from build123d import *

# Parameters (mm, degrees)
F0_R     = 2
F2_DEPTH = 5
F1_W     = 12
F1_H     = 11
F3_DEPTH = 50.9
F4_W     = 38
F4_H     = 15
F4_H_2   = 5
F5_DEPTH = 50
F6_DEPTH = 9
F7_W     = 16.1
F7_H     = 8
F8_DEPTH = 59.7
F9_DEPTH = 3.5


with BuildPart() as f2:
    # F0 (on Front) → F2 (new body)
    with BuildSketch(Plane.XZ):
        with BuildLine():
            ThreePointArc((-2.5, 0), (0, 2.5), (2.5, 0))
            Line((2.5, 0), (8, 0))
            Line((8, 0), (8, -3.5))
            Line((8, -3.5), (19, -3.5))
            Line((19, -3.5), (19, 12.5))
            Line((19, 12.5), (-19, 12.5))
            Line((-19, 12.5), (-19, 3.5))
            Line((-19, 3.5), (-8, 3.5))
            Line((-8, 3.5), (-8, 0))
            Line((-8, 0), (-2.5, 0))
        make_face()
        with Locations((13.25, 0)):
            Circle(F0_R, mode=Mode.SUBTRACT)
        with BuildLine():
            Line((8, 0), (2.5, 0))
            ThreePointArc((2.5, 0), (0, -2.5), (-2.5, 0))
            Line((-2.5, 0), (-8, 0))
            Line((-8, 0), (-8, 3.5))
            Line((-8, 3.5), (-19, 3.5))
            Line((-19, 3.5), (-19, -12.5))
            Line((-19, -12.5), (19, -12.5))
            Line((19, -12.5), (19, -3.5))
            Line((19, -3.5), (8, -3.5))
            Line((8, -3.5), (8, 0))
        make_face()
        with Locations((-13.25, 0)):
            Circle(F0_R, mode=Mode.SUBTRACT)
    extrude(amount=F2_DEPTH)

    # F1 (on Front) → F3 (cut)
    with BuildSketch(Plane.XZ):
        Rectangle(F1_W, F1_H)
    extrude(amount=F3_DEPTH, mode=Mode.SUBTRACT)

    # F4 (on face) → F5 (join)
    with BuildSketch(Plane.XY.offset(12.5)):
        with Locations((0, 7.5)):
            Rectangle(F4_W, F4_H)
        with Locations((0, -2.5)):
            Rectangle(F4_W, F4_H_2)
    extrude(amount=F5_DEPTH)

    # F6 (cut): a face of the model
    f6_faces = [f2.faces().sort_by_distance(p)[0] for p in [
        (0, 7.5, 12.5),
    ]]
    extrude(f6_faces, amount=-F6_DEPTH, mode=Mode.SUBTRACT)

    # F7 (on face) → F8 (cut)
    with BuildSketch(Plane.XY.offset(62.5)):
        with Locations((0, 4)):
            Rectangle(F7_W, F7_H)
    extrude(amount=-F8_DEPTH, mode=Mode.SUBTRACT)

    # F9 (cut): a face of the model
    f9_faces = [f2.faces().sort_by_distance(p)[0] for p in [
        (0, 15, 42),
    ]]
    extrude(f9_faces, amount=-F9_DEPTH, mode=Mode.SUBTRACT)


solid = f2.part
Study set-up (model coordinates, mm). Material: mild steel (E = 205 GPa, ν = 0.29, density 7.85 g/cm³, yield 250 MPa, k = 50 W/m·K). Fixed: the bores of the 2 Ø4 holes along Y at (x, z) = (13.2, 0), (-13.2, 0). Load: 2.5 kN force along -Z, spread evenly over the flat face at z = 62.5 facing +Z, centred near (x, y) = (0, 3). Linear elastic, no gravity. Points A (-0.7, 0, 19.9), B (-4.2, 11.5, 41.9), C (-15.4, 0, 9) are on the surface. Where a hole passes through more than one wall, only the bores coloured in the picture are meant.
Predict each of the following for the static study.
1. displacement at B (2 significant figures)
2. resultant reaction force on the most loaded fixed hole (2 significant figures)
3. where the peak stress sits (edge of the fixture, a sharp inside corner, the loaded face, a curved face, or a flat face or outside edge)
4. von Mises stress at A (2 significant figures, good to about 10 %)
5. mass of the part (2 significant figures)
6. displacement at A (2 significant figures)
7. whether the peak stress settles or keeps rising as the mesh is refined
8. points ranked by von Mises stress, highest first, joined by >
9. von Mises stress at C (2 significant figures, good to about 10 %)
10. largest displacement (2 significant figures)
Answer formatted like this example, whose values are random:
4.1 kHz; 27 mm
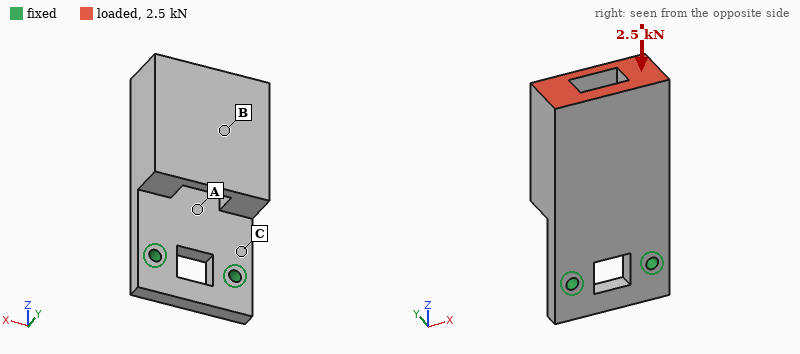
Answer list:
0.16 mm; 1.3 kN; edge of the fixture; 70 MPa; 200 g; 0.045 mm; keeps rising; C > A > B; 130 MPa; 0.25 mm
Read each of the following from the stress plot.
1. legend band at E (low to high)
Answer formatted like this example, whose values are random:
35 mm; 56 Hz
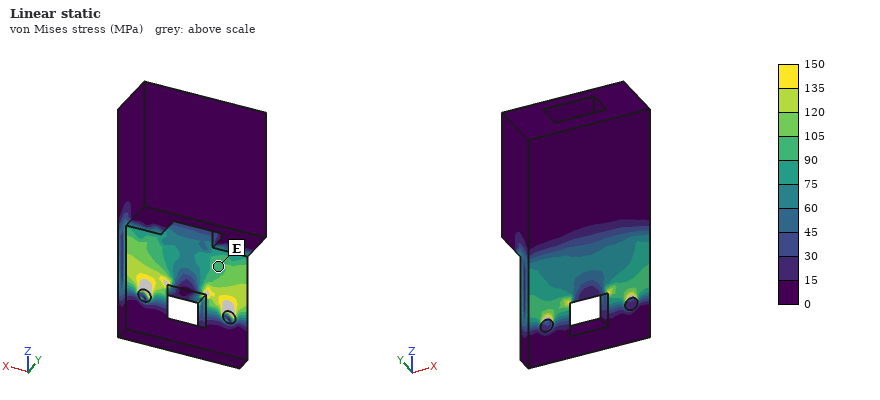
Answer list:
90 to 105 MPa
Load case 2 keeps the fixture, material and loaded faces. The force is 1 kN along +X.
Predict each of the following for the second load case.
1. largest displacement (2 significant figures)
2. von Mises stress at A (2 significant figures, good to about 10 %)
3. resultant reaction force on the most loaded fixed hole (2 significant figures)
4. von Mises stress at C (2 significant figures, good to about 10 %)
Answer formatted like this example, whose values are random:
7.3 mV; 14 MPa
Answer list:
27 µm; 21 MPa; 2.3 kN; 35 MPa
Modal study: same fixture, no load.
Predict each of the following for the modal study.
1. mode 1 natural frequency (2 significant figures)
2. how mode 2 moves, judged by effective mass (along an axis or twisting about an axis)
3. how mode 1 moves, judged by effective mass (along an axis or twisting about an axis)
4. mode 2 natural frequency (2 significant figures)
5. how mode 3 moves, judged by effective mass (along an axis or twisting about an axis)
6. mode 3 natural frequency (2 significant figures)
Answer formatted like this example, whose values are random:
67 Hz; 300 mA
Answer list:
620 Hz; along X; along Y; 2800 Hz; along X; 4200 Hz
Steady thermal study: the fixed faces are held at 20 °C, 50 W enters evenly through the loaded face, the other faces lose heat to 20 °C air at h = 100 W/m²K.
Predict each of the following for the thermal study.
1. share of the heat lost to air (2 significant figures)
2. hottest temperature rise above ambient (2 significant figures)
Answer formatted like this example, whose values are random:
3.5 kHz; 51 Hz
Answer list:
79 %; 85 K
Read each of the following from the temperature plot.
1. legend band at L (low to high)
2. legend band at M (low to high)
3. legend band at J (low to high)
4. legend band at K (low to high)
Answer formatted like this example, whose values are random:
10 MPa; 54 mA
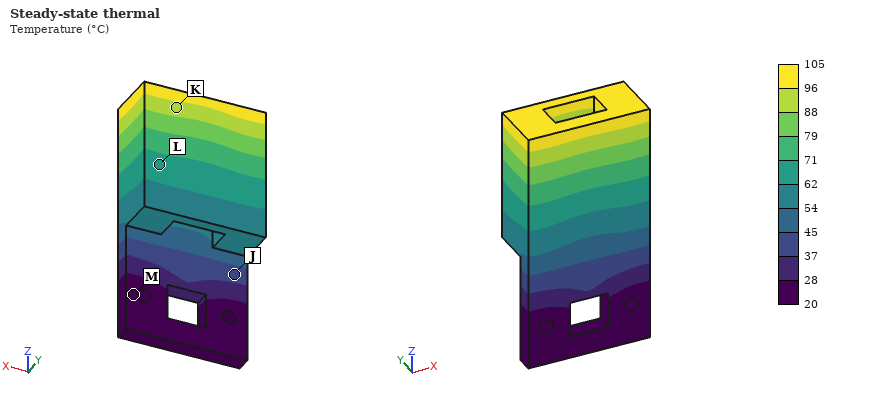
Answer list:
62 to 71 °C; 20 to 28 °C; 37 to 45 °C; 88 to 96 °C
